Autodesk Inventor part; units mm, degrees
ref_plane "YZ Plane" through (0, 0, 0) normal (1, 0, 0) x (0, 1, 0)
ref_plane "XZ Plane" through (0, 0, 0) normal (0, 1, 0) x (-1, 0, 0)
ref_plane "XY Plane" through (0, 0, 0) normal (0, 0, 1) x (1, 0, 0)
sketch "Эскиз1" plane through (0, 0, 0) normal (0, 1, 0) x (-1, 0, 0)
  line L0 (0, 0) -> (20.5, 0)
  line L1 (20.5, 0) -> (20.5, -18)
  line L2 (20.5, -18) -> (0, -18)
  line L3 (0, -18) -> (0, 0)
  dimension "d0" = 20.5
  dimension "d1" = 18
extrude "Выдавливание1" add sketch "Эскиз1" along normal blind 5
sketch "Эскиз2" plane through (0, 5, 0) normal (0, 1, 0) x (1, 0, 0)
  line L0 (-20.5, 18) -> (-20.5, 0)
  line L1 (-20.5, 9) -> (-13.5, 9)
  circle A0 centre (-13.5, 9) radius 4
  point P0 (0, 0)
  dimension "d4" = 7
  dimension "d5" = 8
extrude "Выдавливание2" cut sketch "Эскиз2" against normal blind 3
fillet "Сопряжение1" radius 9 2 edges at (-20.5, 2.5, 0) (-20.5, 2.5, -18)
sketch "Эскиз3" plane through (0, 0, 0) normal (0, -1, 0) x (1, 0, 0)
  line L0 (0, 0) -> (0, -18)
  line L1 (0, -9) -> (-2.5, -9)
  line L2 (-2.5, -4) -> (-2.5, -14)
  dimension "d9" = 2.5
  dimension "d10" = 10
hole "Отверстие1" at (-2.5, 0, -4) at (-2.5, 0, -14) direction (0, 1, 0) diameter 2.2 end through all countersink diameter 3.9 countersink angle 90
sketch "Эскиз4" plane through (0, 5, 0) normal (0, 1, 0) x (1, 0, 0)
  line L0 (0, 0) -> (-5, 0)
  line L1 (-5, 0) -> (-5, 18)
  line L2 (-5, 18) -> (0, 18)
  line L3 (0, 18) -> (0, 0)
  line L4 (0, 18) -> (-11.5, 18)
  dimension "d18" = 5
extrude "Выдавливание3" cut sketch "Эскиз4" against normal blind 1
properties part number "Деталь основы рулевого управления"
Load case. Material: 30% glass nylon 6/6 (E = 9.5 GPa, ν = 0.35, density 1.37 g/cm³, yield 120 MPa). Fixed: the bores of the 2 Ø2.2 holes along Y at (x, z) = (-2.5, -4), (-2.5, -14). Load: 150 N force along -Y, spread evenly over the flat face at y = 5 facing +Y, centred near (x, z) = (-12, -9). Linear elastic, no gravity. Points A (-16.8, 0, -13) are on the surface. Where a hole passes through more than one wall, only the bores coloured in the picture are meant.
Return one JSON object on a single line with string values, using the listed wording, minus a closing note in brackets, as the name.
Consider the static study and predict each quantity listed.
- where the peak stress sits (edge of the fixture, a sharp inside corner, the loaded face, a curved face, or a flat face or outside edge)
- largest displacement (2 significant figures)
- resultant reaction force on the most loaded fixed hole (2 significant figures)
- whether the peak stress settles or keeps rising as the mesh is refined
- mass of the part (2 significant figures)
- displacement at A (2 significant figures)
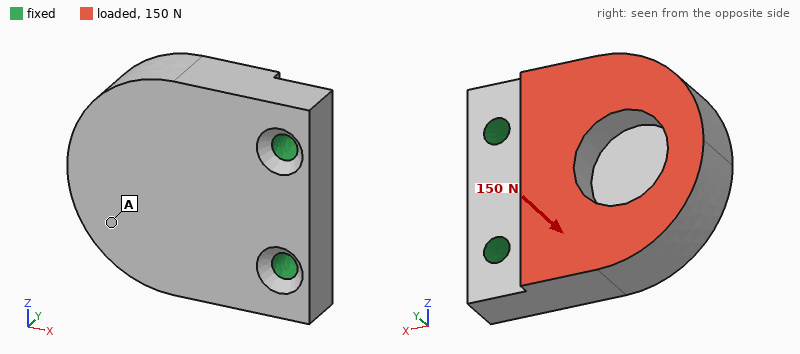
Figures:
{"where the peak stress sits": "edge of the fixture", "largest displacement": "0.14 mm", "resultant reaction force on the most loaded fixed hole": "75 N", "whether the peak stress settles or keeps rising as the mesh is refined": "keeps rising", "mass of the part": "1.9 g", "displacement at A": "0.10 mm"}
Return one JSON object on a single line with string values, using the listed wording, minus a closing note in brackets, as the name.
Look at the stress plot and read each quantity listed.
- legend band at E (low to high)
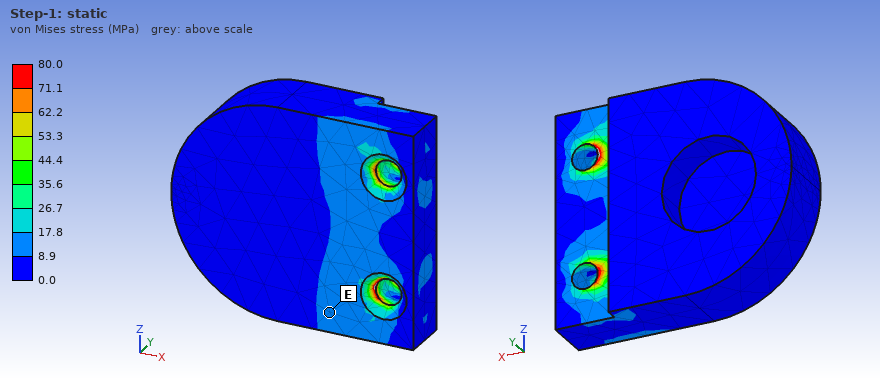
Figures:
{"legend band at E": "8.9 to 17.8 MPa"}
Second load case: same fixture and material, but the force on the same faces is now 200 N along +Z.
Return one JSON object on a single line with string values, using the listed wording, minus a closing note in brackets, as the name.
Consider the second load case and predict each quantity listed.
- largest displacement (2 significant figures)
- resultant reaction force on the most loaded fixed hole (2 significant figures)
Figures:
{"largest displacement": "35 µm", "resultant reaction force on the most loaded fixed hole": "180 N"}
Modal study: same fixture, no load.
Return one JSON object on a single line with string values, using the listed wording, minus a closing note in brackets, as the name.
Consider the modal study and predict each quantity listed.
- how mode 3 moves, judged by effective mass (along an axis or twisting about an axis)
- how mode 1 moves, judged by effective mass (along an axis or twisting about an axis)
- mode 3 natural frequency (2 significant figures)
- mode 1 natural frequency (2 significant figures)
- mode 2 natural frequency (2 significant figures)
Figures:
{"how mode 3 moves, judged by effective mass": "along Z", "how mode 1 moves, judged by effective mass": "along Y", "mode 3 natural frequency": "15 kHz", "mode 1 natural frequency": "5500 Hz", "mode 2 natural frequency": "13 kHz"}
